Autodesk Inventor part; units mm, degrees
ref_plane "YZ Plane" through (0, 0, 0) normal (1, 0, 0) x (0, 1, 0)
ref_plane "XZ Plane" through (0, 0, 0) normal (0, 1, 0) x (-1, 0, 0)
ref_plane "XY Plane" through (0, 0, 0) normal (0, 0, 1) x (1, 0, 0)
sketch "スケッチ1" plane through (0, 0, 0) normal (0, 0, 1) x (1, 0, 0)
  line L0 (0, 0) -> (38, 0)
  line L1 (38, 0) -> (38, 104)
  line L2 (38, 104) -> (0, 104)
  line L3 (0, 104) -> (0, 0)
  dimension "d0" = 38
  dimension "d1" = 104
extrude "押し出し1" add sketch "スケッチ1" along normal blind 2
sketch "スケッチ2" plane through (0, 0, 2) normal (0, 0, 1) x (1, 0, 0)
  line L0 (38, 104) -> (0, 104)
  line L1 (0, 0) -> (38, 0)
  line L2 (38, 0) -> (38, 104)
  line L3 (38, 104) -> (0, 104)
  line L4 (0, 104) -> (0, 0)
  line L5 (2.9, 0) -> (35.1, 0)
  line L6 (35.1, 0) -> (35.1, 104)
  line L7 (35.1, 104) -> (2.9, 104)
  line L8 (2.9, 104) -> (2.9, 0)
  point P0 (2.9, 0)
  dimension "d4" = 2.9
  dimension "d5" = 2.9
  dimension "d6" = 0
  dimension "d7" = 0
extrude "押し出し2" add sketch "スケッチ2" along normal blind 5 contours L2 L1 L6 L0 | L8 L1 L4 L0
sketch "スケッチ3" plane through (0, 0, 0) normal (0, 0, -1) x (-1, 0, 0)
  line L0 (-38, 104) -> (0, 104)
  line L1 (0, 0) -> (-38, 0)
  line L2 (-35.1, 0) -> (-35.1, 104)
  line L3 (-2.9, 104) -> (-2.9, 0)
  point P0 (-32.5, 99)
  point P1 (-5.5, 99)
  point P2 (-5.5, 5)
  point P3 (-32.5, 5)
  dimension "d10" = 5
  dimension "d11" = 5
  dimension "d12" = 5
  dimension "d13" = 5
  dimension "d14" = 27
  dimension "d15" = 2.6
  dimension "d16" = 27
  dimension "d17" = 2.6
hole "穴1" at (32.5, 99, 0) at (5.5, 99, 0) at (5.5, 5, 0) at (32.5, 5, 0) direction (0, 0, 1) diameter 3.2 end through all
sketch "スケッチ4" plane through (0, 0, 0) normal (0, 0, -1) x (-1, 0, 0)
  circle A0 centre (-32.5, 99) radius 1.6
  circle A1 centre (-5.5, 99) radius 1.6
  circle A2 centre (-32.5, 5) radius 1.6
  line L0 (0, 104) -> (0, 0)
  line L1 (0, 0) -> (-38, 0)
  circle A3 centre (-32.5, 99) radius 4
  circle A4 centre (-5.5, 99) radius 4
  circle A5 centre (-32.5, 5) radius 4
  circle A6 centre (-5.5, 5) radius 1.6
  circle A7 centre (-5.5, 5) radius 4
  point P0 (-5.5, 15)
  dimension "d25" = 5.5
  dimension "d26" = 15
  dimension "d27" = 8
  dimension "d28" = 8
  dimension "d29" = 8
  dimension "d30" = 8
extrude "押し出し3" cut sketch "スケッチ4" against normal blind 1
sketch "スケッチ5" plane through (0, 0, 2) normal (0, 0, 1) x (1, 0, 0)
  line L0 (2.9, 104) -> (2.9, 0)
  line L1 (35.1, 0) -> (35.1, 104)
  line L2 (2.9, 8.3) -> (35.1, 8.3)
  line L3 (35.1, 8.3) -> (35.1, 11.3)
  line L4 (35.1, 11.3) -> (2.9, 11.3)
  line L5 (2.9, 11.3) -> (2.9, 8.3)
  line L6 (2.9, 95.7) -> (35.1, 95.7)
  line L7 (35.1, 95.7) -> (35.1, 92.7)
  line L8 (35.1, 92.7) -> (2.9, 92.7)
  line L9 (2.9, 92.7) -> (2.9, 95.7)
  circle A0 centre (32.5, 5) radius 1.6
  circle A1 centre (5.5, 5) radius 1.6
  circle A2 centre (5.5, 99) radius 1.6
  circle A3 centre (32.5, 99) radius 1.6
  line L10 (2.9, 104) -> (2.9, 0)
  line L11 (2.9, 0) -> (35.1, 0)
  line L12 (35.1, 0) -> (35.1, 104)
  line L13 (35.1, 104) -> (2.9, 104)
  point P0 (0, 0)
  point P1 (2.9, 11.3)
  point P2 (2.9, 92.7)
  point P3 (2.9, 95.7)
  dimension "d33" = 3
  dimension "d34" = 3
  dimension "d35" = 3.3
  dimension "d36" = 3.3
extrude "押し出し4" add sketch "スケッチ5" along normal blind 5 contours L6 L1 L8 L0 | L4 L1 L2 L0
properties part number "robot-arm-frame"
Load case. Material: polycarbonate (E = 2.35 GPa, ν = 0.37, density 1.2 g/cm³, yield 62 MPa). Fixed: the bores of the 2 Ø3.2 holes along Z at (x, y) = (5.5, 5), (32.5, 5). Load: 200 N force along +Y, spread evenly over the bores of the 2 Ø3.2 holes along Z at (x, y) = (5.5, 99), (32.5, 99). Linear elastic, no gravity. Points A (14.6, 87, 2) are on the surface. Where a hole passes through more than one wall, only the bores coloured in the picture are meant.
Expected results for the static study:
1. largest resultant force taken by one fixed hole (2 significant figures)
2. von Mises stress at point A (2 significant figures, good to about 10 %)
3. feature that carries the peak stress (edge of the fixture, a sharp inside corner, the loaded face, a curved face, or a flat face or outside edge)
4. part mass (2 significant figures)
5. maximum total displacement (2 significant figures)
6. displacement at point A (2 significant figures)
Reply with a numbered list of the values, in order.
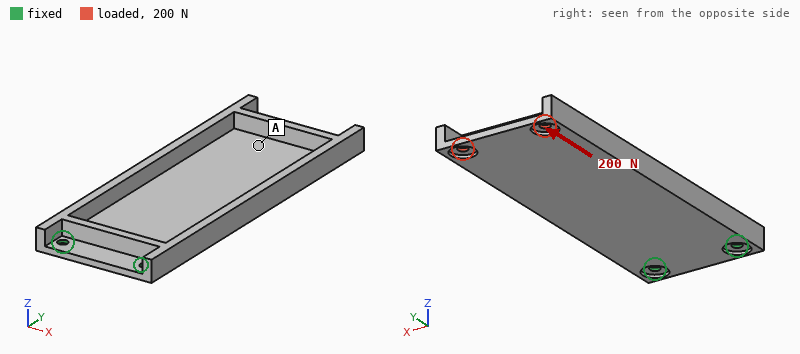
1. 100 N
2. 1.6 MPa
3. the loaded face
4. 14 g
5. 0.64 mm
6. 0.44 mm
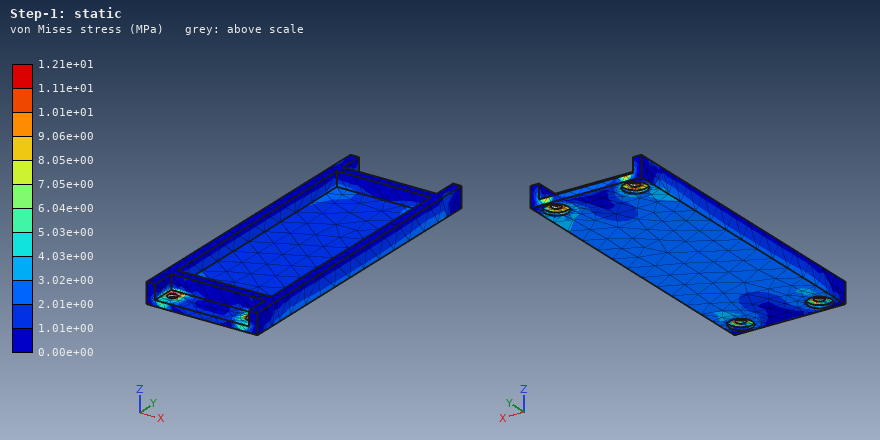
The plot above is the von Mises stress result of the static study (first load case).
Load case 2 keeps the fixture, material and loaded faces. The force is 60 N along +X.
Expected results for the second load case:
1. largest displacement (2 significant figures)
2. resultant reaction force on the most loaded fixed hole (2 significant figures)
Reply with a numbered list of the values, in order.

1. 1.2 mm
2. 200 N
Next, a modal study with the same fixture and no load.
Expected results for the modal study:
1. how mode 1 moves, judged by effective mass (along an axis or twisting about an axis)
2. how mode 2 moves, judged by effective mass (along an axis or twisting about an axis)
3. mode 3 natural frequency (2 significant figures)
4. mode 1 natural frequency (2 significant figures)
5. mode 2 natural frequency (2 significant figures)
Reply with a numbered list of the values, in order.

1. along Z
2. twisting about Y
3. 640 Hz
4. 72 Hz
5. 260 Hz
